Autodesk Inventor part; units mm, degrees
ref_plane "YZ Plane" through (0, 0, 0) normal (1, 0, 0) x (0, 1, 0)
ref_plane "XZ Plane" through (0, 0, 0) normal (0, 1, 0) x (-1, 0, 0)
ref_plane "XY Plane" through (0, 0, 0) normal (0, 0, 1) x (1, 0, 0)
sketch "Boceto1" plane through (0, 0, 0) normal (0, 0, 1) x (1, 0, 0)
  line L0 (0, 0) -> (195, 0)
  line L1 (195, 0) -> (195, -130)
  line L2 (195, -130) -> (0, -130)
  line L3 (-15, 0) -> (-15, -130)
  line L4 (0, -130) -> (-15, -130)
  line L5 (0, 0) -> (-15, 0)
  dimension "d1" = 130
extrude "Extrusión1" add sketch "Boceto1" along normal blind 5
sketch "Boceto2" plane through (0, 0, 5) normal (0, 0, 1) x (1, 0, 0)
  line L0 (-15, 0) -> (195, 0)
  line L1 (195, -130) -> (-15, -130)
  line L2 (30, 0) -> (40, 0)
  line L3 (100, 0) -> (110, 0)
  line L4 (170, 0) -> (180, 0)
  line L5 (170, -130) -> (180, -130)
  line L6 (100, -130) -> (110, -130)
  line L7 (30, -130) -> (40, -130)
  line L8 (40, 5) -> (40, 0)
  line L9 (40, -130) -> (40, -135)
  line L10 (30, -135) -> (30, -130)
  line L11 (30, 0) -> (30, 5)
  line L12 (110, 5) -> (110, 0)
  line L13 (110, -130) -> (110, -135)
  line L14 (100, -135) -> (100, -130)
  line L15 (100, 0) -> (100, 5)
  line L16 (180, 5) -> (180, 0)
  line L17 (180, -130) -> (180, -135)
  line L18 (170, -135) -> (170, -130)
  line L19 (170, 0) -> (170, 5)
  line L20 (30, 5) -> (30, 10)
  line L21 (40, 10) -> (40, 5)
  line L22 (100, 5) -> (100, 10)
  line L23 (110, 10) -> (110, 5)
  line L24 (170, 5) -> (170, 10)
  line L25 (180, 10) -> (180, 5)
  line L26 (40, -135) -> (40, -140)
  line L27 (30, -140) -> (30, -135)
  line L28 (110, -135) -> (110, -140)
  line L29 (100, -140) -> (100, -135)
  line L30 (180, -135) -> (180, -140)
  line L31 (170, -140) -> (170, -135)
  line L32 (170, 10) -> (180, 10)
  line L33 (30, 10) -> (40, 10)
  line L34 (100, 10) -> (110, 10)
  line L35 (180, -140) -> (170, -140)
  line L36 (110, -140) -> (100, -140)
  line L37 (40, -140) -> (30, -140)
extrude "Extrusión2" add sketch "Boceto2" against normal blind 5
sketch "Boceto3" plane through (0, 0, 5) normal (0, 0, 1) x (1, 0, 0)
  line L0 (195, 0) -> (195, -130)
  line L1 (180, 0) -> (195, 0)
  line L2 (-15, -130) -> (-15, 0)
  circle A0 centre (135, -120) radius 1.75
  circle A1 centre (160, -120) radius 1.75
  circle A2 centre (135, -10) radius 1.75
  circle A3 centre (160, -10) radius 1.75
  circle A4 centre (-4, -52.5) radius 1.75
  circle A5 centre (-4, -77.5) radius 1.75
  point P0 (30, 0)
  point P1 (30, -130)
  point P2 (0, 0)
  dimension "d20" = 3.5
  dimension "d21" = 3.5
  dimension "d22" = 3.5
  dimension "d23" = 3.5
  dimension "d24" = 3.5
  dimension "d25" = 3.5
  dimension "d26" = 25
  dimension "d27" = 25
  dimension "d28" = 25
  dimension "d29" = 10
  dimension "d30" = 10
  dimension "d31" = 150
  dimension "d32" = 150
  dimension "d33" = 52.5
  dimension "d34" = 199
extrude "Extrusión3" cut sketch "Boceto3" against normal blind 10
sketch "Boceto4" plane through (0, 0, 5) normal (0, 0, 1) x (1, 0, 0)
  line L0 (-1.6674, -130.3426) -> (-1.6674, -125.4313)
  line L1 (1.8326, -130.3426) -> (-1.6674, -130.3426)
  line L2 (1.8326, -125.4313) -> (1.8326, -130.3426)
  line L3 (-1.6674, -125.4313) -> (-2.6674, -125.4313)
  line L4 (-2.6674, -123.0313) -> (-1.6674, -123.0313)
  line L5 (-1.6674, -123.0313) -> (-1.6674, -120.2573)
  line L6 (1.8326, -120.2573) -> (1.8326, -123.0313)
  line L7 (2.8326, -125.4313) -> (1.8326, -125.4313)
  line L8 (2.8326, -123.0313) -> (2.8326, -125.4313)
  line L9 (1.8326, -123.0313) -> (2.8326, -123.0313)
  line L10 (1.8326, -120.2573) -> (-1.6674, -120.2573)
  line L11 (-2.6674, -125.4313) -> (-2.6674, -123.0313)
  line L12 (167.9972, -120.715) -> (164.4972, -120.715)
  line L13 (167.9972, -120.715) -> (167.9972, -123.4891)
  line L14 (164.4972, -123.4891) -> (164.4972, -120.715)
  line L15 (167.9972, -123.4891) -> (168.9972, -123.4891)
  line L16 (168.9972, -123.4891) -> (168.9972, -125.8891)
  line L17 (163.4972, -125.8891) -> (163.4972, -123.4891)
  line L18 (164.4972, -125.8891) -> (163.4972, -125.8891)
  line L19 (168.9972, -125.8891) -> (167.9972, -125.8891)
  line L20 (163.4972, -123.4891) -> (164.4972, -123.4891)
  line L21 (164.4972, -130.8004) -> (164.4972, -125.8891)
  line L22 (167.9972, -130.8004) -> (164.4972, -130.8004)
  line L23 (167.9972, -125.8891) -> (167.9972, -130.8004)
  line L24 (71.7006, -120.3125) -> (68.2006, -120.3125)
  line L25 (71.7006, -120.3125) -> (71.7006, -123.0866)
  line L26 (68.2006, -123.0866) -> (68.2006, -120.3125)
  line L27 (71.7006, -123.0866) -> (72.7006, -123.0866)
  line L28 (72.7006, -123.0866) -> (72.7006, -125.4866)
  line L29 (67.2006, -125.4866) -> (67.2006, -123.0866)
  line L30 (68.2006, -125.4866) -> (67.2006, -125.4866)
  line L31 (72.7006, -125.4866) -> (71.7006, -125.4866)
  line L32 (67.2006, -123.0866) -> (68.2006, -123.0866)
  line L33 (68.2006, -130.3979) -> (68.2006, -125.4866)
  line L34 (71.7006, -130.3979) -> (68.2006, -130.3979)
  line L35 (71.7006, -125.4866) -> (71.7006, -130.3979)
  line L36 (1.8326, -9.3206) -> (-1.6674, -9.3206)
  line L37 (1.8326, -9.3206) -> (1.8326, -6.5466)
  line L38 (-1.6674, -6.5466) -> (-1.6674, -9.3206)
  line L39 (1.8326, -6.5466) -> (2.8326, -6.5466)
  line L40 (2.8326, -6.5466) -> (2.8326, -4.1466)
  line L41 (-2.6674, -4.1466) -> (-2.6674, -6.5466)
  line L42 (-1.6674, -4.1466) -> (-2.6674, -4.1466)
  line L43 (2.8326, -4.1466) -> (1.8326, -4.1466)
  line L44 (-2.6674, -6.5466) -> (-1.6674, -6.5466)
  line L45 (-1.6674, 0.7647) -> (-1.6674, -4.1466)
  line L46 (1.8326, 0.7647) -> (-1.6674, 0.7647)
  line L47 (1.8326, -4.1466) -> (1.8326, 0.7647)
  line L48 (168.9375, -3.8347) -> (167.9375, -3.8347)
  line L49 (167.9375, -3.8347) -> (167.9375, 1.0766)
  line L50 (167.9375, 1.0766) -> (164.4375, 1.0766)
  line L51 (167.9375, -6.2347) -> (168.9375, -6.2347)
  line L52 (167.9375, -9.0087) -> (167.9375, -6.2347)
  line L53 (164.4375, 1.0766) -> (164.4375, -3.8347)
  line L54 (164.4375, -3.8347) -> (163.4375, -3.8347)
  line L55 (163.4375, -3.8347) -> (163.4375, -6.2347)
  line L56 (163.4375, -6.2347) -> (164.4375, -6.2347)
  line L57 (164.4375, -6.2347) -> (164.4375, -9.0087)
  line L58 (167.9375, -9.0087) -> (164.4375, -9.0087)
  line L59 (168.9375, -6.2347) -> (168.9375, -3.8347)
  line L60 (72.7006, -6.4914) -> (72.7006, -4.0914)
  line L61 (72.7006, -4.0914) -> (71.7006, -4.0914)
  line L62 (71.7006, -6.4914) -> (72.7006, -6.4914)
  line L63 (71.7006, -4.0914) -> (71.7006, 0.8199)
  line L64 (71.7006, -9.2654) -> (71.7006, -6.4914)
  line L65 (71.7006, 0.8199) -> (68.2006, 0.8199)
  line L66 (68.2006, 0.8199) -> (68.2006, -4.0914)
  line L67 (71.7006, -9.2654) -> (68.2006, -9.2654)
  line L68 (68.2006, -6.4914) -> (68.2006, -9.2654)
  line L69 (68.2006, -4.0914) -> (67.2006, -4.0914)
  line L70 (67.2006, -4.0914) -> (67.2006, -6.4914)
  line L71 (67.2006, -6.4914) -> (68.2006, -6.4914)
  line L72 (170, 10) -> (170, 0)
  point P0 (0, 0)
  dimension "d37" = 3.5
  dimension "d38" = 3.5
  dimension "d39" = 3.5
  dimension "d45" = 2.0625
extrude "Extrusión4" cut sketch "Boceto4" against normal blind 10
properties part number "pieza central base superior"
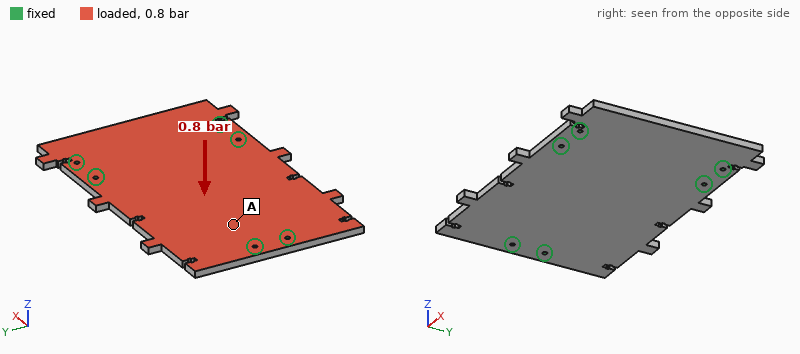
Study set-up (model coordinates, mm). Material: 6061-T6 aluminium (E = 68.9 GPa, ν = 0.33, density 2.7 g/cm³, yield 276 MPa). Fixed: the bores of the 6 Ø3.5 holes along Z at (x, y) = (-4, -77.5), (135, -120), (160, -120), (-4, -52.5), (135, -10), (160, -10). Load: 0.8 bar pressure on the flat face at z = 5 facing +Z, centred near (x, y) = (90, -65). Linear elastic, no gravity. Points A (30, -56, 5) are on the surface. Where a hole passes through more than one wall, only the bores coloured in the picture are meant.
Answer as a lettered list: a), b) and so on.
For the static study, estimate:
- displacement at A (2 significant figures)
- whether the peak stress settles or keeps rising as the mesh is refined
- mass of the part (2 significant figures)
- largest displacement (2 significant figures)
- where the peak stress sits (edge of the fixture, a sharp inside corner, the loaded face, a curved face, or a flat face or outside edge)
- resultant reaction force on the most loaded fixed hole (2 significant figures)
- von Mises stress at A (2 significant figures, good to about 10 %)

a) 0.11 mm
b) keeps rising
c) 370 g
d) 0.27 mm
e) edge of the fixture
f) 520 N
g) 14 MPa
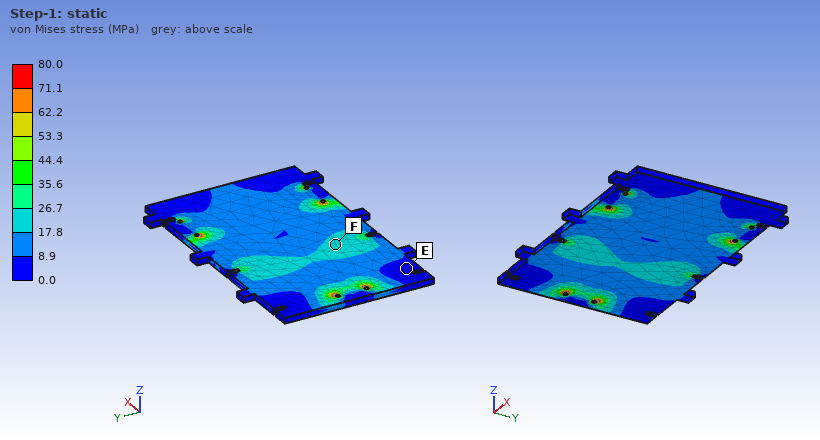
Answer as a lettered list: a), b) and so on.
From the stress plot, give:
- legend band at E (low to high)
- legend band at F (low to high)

a) 0.0 to 8.9 MPa
b) 17.8 to 26.7 MPa
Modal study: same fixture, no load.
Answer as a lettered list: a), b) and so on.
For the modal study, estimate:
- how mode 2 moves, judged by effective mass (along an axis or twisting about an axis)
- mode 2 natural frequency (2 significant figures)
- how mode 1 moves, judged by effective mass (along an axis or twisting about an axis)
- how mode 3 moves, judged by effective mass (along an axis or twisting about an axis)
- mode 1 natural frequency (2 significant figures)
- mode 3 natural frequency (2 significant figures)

a) twisting about X
b) 1000 Hz
c) along Z
d) along Z
e) 950 Hz
f) 1500 Hz
